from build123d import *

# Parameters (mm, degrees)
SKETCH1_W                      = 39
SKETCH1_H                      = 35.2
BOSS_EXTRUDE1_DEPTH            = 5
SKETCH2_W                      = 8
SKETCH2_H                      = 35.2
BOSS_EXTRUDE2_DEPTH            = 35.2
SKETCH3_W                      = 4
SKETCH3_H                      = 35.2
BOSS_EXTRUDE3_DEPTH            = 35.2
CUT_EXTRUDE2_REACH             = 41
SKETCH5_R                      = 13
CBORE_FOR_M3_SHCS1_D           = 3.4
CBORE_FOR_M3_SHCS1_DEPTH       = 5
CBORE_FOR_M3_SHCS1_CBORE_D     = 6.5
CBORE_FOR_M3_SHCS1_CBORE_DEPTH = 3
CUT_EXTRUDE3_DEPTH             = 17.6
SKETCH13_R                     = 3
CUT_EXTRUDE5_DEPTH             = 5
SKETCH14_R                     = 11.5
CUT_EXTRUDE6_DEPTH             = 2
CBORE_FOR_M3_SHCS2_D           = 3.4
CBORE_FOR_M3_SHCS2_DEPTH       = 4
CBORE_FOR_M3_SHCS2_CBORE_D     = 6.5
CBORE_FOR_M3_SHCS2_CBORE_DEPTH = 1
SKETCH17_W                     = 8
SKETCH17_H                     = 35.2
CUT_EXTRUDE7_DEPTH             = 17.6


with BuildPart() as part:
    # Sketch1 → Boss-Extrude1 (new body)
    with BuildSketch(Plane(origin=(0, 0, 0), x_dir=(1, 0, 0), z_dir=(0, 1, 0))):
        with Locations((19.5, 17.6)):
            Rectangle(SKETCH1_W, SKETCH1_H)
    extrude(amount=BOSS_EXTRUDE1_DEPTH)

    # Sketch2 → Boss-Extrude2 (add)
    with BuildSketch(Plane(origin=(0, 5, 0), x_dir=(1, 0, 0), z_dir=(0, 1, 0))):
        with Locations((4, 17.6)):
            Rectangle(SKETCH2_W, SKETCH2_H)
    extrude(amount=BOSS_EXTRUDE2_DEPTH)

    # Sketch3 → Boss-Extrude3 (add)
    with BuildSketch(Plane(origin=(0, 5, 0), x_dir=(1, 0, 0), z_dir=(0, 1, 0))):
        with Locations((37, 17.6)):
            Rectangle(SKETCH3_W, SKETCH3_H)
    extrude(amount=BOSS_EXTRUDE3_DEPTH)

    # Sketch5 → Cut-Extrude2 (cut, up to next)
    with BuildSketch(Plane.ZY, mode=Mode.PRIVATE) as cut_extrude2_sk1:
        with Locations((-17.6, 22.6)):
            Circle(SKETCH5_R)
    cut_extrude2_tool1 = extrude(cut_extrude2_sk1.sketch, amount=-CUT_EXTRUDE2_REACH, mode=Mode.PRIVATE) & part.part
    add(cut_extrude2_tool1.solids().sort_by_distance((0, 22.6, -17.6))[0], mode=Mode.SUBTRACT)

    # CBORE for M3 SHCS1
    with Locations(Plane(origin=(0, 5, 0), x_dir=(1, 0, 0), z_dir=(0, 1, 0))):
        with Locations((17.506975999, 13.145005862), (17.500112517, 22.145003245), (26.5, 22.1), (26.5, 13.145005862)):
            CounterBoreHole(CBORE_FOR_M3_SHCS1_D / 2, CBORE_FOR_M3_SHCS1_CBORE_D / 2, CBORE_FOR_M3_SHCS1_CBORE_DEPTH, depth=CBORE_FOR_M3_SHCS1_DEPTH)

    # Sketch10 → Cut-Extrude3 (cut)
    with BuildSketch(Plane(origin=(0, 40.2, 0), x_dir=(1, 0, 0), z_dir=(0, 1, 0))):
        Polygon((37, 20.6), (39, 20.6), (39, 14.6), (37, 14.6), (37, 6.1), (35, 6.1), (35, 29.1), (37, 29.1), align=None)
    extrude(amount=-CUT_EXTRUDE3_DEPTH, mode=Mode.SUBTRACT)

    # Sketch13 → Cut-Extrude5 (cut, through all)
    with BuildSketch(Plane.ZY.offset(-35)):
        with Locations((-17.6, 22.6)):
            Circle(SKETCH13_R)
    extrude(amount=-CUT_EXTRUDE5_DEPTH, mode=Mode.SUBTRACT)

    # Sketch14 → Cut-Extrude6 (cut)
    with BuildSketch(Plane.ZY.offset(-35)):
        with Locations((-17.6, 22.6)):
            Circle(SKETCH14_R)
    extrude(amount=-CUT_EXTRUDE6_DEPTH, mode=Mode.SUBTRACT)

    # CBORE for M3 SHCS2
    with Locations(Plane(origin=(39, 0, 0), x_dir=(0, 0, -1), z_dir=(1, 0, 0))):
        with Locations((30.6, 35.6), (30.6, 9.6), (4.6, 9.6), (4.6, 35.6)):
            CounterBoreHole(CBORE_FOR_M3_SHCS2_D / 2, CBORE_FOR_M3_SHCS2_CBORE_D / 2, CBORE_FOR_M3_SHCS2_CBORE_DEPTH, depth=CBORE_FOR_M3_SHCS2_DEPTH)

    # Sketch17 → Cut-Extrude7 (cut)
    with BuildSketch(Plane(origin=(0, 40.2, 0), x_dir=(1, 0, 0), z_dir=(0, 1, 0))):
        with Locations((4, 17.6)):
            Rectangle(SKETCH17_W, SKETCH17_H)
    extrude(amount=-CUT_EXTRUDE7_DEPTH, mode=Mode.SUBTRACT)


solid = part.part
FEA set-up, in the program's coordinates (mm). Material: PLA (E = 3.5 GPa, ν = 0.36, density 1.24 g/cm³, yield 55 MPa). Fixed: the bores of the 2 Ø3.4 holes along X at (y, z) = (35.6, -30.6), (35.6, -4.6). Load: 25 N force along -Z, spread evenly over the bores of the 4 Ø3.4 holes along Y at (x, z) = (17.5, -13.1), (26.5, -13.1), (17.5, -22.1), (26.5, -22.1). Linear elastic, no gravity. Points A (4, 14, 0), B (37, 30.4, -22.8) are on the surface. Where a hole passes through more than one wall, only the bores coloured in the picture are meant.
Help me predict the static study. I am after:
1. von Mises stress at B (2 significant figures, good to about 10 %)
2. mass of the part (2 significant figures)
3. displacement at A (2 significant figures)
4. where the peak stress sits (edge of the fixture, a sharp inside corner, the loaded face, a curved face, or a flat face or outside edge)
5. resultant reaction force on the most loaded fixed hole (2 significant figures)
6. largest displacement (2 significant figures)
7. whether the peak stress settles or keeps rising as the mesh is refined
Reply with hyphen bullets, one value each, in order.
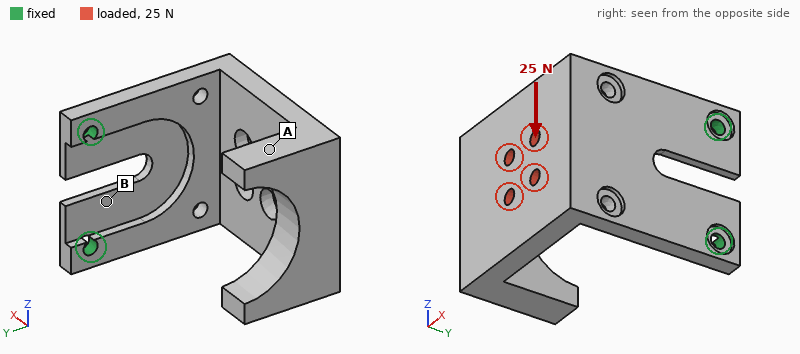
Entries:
- 2.1 MPa
- 15 g
- 0.62 mm
- edge of the fixture
- 31 N
- 0.69 mm
- keeps rising
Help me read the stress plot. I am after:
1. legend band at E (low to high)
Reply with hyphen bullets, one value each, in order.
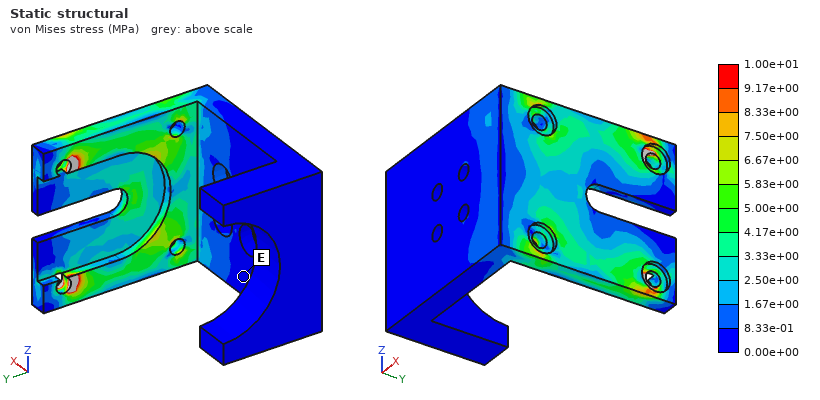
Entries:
- 0.00e+00 to 8.33e-01 MPa
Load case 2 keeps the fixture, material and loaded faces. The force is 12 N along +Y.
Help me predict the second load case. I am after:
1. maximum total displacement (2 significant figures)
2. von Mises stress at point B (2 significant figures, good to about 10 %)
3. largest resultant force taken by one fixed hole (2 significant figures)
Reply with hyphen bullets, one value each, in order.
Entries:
- 0.77 mm
- 1.6 MPa
- 6.7 N
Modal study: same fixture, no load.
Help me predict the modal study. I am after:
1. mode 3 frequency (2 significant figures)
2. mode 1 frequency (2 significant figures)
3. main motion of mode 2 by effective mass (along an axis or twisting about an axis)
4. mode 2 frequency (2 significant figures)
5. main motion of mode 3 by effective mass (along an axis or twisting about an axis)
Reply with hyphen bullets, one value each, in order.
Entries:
- 480 Hz
- 150 Hz
- along Z
- 260 Hz
- along X
